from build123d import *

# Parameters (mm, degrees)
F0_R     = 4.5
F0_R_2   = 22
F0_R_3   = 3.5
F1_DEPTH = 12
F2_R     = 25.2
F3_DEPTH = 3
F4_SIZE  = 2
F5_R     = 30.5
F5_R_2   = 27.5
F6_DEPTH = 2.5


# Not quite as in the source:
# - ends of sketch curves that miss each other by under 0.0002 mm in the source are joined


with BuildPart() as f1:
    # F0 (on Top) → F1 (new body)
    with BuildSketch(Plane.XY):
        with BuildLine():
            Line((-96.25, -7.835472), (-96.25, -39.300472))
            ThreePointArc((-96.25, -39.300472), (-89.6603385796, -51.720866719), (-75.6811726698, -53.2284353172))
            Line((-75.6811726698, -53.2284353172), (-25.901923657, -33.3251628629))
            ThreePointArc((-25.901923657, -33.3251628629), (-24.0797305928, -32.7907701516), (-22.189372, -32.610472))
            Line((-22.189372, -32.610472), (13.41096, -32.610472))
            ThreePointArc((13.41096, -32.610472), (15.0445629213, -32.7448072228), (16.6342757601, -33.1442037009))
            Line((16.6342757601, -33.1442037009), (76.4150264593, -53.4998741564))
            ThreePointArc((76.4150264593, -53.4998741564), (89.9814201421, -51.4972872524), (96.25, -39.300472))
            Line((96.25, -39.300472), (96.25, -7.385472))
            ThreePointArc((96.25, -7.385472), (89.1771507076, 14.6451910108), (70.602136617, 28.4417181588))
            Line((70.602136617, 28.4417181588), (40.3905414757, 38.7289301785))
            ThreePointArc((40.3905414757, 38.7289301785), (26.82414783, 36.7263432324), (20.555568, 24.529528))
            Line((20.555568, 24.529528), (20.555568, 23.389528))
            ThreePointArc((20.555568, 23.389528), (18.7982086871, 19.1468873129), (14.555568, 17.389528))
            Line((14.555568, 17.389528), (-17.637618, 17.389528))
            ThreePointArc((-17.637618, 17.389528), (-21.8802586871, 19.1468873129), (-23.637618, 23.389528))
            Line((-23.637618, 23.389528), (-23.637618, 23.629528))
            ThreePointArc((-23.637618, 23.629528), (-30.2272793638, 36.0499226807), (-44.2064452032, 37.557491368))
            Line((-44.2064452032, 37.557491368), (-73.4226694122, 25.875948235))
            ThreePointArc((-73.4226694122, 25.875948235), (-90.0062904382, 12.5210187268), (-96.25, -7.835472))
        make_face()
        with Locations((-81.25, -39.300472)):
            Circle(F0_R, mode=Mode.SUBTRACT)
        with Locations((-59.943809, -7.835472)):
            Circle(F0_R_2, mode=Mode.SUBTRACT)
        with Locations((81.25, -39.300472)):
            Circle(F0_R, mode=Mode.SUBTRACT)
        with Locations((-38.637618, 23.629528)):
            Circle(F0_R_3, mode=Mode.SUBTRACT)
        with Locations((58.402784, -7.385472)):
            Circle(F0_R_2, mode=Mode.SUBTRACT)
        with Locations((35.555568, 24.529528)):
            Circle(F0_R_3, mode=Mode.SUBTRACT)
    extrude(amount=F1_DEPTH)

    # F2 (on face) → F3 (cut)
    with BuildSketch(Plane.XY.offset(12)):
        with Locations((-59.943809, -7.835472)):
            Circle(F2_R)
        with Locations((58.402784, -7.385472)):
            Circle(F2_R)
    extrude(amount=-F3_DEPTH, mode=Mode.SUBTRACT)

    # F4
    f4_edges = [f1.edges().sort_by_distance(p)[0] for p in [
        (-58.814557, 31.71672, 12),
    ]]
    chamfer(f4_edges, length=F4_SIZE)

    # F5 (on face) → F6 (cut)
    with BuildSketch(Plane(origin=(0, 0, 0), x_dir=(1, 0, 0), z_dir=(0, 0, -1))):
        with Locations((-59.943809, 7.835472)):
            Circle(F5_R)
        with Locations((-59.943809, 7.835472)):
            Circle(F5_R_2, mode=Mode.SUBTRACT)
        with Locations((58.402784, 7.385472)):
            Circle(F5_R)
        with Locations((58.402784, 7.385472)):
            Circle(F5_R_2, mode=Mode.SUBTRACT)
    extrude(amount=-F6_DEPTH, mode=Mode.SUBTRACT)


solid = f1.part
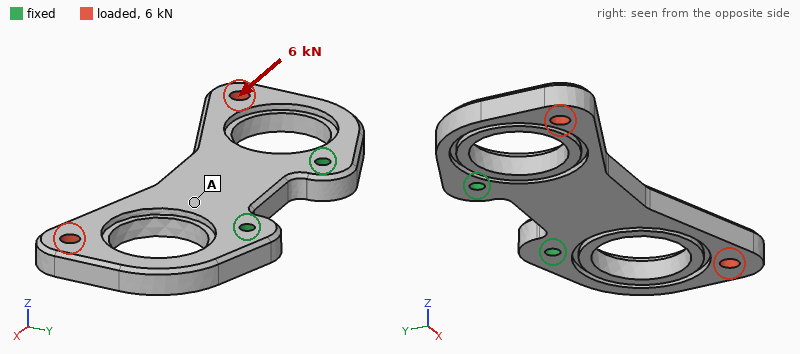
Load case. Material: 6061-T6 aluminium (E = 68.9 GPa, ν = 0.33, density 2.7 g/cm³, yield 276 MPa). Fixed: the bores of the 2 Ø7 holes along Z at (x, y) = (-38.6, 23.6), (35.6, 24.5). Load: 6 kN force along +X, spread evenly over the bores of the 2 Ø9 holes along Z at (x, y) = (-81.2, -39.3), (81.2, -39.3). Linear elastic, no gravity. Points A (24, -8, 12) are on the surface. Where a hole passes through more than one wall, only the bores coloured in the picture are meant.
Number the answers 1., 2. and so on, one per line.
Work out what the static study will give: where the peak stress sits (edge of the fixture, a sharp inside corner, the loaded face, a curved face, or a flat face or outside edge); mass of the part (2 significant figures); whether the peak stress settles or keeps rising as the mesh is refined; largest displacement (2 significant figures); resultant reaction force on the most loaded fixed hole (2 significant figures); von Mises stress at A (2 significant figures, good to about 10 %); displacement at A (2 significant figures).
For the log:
1. edge of the fixture
2. 310 g
3. keeps rising
4. 77 µm
5. 5.6 kN
6. 10 MPa
7. 15 µm
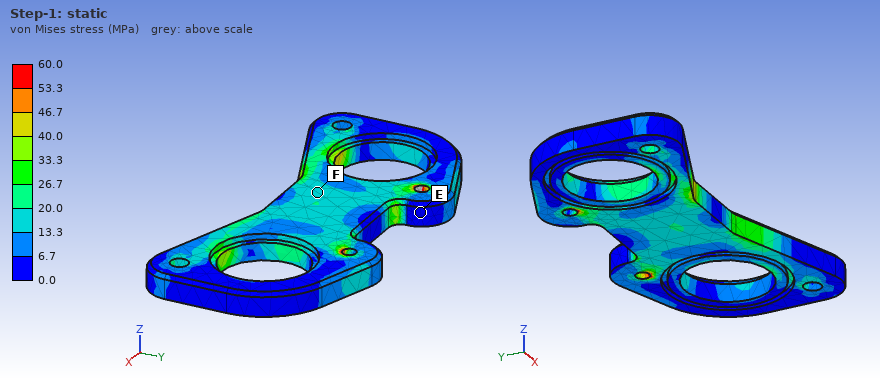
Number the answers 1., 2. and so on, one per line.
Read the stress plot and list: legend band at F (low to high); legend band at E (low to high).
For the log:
1. 13.3 to 20.0 MPa
2. 0.0 to 6.7 MPa
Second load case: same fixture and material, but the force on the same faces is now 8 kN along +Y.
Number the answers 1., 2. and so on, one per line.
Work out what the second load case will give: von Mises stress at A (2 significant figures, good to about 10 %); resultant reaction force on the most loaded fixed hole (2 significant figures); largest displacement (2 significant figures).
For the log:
1. 13 MPa
2. 5.1 kN
3. 0.12 mm
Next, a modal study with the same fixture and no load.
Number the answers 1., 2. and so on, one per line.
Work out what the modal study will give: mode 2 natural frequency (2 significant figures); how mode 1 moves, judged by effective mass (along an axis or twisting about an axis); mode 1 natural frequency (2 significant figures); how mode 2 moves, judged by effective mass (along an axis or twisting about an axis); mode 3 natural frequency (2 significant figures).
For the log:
1. 1200 Hz
2. along Z
3. 1100 Hz
4. twisting about Y
5. 2200 Hz
